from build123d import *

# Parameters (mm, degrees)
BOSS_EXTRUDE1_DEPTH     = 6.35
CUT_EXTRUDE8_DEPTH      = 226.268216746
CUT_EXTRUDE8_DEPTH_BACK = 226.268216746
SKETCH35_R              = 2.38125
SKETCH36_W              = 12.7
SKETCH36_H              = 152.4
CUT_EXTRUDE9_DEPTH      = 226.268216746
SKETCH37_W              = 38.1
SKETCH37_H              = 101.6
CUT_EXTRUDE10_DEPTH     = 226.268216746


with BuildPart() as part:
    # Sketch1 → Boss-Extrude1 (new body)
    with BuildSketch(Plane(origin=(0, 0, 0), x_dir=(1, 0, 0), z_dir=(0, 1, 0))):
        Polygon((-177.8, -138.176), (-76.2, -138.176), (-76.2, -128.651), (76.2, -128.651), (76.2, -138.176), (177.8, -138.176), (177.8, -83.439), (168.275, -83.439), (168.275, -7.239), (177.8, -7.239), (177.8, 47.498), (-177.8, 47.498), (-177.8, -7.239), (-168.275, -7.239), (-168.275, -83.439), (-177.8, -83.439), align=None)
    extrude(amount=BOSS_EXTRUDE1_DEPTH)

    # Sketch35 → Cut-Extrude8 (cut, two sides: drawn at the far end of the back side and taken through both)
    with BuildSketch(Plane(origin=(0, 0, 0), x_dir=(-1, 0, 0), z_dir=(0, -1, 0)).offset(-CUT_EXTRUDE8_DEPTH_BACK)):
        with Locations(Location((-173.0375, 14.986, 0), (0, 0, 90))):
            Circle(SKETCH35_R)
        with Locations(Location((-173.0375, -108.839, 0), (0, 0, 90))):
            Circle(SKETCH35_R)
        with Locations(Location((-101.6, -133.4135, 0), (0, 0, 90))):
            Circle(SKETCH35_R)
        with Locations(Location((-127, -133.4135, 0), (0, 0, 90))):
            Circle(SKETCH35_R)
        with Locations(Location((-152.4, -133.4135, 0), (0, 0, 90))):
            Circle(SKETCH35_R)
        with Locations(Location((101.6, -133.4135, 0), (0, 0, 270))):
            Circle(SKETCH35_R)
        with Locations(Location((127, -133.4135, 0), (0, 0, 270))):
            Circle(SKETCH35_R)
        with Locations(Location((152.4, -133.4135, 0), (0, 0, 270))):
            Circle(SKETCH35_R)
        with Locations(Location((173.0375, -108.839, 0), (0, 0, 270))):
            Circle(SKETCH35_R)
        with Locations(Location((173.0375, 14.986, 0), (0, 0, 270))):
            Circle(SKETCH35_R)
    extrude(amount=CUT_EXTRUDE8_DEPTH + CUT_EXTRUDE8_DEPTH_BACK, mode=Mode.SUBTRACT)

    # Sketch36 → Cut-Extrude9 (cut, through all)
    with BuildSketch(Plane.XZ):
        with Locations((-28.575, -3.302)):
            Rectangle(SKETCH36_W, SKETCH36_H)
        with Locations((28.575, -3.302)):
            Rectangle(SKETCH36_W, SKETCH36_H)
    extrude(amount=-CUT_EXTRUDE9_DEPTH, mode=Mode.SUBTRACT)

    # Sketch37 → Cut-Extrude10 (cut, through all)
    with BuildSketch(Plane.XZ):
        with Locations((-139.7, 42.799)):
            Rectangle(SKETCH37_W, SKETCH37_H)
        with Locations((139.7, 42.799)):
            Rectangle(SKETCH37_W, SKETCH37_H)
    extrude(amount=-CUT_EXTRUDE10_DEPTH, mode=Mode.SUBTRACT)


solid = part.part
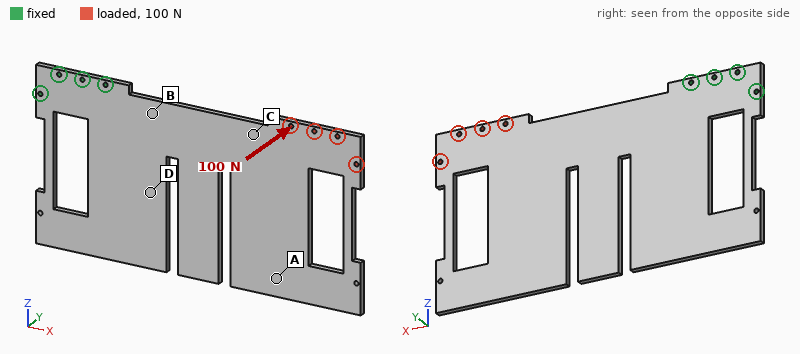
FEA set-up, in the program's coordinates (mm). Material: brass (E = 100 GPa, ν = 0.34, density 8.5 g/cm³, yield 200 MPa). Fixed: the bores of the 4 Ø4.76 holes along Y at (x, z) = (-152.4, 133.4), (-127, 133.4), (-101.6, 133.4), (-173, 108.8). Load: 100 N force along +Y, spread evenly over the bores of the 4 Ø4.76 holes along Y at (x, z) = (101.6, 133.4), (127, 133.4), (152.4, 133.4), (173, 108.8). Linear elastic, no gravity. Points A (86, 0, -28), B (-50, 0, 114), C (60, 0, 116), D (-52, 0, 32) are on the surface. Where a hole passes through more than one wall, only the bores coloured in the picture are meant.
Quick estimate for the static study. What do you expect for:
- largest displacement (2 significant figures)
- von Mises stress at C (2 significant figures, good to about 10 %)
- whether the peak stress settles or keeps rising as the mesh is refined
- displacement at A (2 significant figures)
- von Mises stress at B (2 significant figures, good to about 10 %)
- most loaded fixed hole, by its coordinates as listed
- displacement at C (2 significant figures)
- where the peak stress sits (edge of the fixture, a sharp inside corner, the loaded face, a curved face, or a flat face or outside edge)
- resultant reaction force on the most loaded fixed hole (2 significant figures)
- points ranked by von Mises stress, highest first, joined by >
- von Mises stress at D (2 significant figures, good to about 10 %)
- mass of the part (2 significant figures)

4.4 mm
18 MPa
keeps rising
2.3 mm
42 MPa
(-101.6, 133.4)
1.9 mm
edge of the fixture
580 N
B > C > D > A
11 MPa
2.8 kg
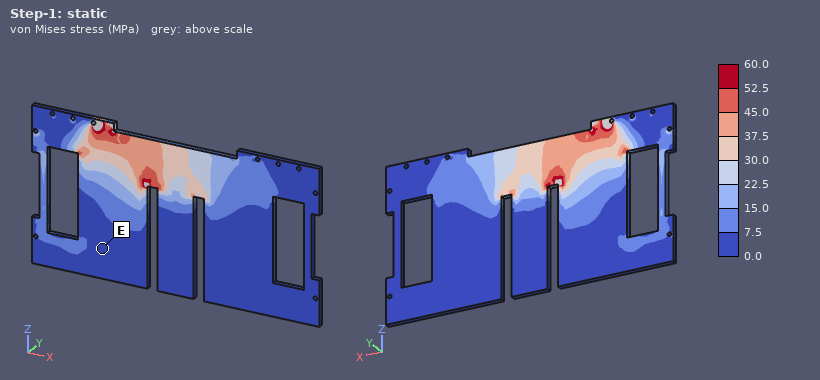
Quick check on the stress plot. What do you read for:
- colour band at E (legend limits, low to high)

0.0 to 7.5 MPa
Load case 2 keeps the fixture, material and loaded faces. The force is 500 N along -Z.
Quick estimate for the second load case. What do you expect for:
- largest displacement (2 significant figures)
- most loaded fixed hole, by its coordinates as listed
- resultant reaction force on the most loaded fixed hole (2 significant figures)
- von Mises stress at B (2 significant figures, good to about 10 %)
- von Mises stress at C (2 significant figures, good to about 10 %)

0.38 mm
(-101.6, 133.4)
2.9 kN
11 MPa
5.9 MPa
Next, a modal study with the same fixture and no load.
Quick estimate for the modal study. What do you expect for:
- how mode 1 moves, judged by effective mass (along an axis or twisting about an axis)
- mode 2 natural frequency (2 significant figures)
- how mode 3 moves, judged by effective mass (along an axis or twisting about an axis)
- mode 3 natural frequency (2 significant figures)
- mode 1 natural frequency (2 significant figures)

along Y
69 Hz
along Y
110 Hz
27 Hz
